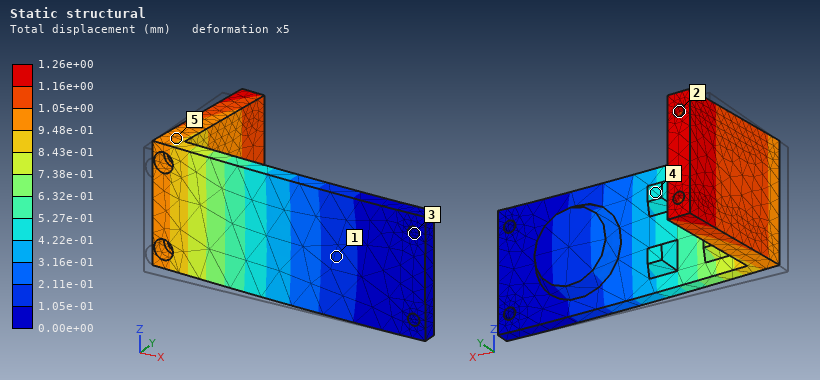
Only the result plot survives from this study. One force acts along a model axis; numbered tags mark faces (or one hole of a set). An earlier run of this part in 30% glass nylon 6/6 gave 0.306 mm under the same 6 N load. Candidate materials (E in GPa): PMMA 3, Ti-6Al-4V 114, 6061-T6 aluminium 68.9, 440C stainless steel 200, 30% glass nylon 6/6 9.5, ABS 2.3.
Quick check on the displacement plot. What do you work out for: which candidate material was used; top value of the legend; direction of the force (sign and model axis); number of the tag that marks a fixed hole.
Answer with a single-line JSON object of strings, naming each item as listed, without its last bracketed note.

{"which candidate material was used": "ABS", "top value of the legend": "1.26e+00 mm", "direction of the force": "+Y", "number of the tag that marks a fixed hole": "3"}
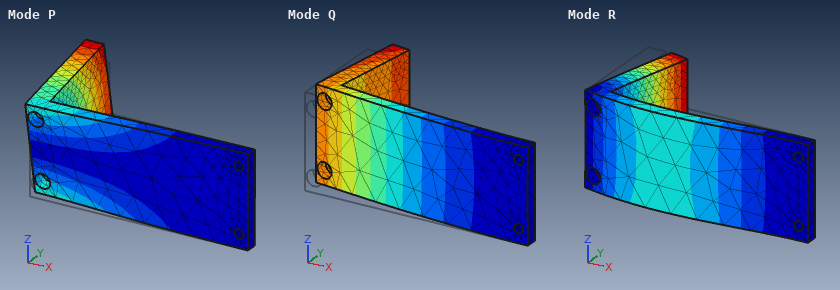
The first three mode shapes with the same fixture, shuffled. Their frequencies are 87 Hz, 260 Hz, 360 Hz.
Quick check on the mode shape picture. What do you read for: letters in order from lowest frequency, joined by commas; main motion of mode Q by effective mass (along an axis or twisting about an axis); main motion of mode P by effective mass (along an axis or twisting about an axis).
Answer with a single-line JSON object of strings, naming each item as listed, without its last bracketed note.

{"letters in order from lowest frequency, joined by commas": "Q, P, R", "main motion of mode Q by effective mass": "along Y", "main motion of mode P by effective mass": "along Z"}
